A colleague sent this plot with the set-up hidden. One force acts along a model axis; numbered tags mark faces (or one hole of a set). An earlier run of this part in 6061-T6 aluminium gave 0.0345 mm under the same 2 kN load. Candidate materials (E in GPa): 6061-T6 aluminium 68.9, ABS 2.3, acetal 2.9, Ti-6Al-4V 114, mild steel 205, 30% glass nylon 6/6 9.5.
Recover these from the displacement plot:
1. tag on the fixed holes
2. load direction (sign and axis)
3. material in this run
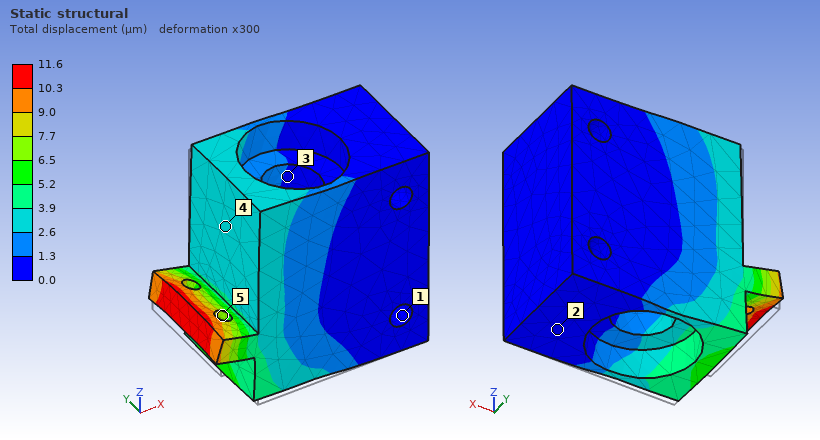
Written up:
1
+Z
mild steel
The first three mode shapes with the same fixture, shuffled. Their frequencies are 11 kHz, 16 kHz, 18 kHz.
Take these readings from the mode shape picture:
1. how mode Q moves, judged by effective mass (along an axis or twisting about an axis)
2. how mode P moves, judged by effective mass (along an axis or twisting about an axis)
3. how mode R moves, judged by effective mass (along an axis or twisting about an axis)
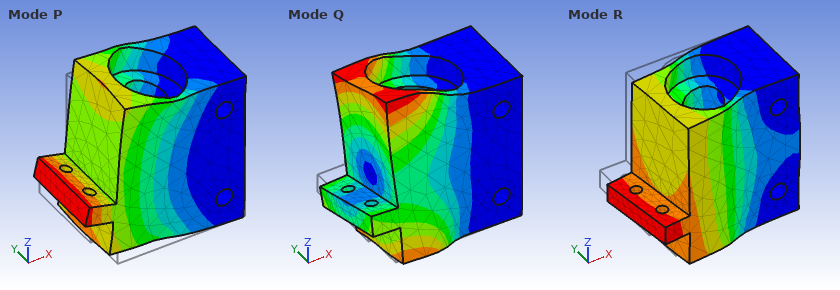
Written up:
twisting about X
along Z
along Y
